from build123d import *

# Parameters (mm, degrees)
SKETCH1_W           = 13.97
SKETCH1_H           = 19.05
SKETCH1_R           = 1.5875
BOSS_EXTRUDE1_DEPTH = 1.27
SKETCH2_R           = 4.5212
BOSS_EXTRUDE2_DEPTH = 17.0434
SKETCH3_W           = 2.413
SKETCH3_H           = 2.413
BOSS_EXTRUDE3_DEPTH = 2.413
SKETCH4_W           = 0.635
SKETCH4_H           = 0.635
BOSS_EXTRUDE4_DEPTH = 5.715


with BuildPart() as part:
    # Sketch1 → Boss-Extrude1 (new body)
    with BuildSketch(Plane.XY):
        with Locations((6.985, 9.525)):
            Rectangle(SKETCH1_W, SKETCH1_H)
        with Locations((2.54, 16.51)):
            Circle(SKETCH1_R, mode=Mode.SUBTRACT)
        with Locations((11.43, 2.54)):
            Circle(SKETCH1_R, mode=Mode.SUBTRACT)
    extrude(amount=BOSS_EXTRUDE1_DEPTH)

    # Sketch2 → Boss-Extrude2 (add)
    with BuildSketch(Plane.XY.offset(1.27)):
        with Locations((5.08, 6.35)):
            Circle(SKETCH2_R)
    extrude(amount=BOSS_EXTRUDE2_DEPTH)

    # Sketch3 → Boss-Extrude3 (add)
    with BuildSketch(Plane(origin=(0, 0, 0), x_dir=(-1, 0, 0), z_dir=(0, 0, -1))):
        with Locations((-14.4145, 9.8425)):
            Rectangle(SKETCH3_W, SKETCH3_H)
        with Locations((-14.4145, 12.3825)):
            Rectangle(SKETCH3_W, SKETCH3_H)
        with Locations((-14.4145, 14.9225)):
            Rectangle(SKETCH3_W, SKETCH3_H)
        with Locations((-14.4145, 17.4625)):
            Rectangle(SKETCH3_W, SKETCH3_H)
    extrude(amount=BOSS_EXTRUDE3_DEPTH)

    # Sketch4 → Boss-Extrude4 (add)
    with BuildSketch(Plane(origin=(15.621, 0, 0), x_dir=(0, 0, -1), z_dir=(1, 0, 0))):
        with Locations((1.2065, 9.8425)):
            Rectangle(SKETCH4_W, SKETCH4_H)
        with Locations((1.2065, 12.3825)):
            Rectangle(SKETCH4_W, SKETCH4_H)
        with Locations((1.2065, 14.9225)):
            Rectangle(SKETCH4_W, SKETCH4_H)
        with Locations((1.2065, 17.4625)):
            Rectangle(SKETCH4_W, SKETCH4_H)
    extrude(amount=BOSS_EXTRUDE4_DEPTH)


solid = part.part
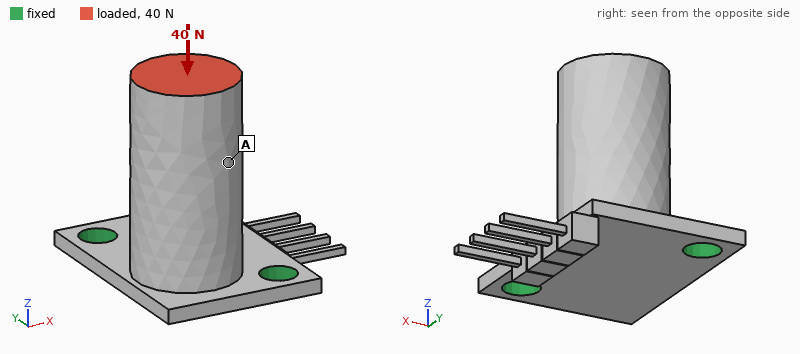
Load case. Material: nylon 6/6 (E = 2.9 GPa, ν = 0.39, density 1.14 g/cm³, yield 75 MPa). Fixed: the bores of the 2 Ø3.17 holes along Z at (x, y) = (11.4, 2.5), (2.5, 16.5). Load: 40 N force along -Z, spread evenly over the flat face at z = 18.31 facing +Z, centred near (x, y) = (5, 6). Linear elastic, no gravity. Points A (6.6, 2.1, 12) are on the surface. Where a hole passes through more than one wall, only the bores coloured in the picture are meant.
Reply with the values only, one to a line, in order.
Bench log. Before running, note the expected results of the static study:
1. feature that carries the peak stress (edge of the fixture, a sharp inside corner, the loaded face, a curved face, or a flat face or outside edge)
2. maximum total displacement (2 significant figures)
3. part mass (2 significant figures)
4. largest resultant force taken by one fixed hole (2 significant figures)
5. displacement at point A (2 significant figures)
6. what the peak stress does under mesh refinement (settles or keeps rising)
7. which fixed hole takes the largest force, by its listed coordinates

edge of the fixture
0.39 mm
1.7 g
25 N
0.23 mm
keeps rising
(11.4, 2.5)
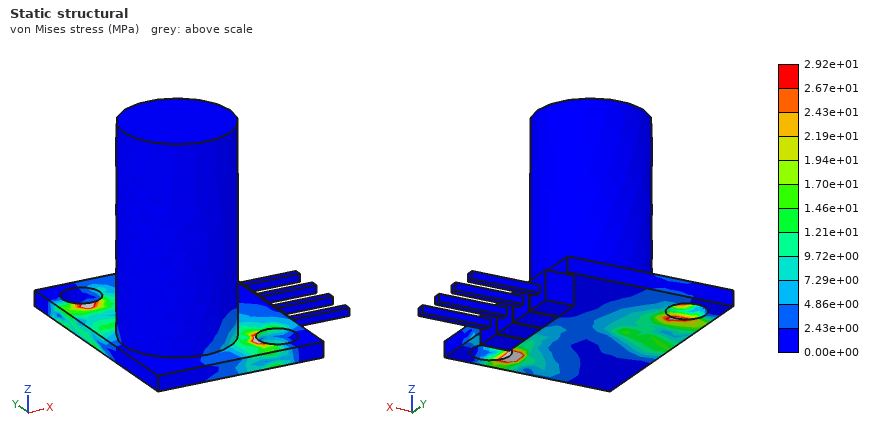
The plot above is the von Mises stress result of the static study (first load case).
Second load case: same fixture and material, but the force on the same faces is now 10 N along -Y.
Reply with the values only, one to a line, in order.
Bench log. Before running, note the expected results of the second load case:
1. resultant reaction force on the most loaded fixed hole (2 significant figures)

13 N
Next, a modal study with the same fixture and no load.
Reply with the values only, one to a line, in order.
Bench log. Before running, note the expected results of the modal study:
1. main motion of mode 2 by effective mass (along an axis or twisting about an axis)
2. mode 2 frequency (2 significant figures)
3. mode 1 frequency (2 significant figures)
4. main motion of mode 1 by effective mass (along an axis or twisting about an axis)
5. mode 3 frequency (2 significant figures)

along Y
2000 Hz
930 Hz
along X
2500 Hz
